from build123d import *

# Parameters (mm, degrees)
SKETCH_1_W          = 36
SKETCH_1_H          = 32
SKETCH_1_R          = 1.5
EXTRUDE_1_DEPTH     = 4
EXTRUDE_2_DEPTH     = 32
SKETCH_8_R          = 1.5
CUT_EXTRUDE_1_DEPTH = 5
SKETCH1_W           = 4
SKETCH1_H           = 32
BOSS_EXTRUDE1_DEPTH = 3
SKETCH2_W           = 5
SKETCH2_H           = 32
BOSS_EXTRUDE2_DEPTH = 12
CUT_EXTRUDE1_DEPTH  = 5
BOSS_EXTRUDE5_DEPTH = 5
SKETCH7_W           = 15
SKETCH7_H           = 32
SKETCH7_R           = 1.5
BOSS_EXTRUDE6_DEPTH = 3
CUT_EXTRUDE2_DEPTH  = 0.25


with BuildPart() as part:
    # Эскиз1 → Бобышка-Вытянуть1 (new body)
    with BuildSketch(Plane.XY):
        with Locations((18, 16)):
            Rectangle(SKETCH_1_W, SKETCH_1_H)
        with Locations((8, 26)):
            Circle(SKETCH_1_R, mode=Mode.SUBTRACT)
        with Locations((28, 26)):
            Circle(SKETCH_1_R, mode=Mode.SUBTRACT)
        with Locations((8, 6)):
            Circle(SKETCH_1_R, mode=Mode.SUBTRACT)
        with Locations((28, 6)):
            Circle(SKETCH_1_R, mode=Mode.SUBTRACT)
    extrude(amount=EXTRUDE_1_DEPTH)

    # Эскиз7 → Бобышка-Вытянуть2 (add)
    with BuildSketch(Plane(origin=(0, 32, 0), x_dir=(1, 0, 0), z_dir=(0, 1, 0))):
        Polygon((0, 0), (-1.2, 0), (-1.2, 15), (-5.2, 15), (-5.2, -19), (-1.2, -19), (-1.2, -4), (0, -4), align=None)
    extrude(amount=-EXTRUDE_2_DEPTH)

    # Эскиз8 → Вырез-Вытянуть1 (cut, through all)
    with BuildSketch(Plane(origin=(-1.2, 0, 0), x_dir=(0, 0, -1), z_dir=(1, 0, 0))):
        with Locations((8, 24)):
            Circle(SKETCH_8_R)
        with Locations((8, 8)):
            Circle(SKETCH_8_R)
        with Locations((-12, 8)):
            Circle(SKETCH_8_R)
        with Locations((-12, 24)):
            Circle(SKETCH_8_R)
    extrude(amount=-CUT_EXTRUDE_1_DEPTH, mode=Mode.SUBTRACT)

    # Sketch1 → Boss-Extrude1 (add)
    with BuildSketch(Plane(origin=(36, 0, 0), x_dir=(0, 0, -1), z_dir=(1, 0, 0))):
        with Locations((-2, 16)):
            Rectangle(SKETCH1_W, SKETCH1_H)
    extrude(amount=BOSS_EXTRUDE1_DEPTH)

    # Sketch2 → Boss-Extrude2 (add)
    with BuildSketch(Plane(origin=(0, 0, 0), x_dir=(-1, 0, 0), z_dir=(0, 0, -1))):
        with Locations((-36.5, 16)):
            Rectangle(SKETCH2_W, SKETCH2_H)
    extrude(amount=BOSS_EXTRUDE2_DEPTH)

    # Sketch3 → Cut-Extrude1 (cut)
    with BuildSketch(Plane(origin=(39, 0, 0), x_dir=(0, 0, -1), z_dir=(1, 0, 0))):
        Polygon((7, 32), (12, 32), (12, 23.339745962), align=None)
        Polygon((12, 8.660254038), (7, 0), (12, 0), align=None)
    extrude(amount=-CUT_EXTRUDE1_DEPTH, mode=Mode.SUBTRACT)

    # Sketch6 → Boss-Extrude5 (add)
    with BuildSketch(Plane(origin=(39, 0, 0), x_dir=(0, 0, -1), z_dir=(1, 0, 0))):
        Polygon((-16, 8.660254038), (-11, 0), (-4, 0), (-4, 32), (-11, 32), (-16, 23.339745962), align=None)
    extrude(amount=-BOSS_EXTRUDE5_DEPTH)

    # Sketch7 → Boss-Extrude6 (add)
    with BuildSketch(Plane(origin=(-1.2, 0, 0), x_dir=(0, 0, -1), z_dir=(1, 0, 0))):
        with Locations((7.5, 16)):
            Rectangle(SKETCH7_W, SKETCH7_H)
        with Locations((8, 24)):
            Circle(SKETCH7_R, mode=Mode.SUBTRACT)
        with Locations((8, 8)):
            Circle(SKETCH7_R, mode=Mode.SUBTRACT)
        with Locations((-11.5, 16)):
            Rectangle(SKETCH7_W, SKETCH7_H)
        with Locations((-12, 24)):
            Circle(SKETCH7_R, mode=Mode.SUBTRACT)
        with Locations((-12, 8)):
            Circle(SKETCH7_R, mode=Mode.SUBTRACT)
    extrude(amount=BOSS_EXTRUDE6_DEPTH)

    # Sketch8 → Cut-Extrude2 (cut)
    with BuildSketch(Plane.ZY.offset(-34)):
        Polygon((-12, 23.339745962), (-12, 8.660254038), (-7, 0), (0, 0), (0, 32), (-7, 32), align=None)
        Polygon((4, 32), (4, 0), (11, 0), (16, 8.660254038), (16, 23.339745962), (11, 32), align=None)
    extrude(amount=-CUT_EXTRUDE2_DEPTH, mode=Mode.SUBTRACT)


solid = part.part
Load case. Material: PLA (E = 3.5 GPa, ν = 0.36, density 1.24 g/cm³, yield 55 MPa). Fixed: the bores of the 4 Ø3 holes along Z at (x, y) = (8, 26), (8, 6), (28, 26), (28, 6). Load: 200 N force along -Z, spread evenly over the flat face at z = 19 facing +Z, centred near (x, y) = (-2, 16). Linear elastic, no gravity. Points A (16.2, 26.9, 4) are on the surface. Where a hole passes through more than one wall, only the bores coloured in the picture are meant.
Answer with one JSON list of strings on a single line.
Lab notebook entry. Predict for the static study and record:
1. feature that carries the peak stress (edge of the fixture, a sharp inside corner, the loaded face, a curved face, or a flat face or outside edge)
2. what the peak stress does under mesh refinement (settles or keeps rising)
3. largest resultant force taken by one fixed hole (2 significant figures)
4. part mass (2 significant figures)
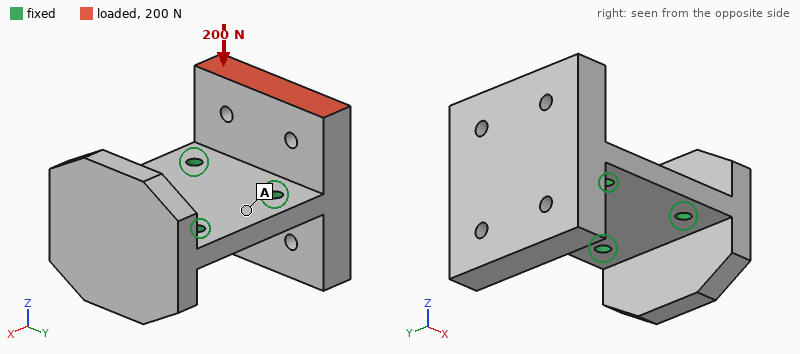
["edge of the fixture", "keeps rising", "110 N", "19 g"]
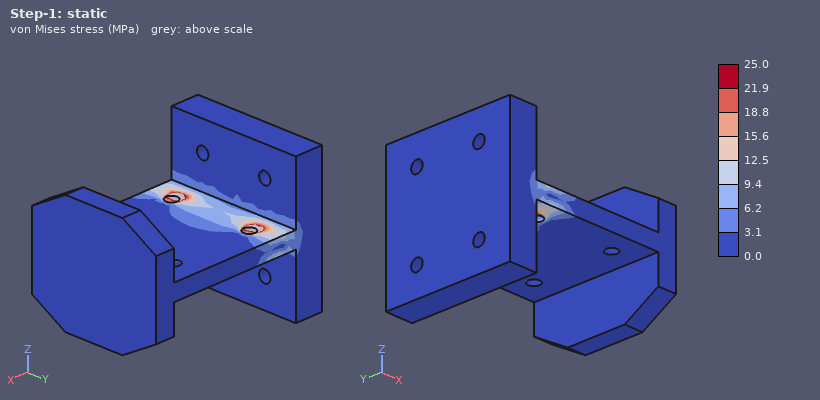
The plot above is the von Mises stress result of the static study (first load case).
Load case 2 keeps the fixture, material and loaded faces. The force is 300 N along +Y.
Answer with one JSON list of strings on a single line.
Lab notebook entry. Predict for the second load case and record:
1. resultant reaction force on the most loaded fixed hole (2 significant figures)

["300 N"]
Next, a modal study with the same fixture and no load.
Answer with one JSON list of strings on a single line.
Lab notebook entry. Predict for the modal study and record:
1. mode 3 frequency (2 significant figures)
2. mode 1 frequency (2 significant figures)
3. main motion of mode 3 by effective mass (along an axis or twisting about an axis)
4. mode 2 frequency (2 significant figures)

["3100 Hz", "1200 Hz", "twisting about X", "2200 Hz"]
